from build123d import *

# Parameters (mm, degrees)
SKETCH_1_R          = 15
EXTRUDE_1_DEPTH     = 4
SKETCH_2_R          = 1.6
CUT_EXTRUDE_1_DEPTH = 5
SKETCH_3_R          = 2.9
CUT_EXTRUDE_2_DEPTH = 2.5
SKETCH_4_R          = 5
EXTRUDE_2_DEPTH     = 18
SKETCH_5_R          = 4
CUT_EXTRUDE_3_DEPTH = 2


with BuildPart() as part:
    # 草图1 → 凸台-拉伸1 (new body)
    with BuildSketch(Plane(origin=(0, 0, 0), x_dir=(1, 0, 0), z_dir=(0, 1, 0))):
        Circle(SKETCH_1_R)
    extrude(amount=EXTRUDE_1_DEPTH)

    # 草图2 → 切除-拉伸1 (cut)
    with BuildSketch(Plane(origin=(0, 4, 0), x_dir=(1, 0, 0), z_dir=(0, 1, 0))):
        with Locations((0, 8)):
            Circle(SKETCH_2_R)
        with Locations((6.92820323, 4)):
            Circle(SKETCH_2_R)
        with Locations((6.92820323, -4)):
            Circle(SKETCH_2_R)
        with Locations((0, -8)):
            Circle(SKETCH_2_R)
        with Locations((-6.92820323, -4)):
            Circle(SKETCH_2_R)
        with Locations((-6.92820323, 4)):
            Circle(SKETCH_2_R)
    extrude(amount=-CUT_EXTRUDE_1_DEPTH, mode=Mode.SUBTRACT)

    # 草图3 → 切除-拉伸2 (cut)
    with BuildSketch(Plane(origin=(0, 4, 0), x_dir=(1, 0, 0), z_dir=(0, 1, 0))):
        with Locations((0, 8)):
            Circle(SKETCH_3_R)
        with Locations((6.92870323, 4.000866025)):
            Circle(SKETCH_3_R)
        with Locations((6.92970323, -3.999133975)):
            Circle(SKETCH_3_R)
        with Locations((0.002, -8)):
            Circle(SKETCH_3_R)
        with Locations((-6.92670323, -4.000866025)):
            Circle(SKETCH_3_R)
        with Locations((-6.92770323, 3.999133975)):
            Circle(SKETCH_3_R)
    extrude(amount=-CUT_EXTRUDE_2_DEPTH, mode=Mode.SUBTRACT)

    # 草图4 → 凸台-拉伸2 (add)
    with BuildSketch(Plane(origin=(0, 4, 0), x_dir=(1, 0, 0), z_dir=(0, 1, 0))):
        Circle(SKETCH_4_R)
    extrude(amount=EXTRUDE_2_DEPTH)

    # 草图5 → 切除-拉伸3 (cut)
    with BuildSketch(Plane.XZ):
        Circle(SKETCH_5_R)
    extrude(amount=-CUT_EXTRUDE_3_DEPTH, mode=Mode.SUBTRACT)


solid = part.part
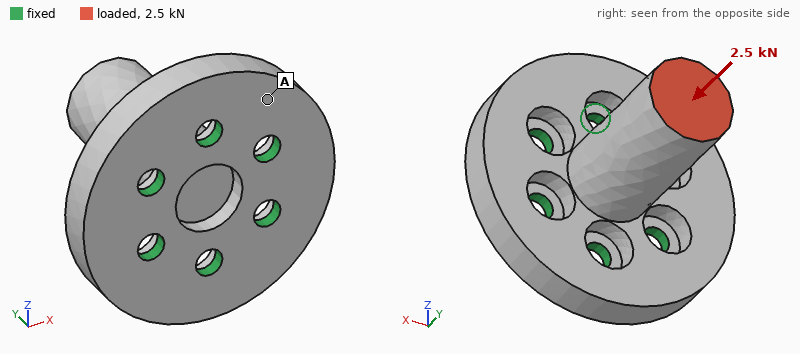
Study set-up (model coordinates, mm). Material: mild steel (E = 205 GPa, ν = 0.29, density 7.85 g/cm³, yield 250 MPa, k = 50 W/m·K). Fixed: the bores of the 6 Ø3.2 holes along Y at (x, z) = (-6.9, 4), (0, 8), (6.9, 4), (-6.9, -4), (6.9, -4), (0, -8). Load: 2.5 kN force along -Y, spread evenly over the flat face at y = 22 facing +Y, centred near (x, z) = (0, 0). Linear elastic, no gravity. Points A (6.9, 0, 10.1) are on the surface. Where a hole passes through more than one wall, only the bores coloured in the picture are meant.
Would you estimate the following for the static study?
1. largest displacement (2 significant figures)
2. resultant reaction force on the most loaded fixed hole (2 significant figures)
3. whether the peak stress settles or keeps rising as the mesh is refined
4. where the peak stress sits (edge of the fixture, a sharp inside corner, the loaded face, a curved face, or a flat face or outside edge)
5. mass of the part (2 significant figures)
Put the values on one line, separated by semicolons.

5.2 µm; 520 N; keeps rising; edge of the fixture; 29 g
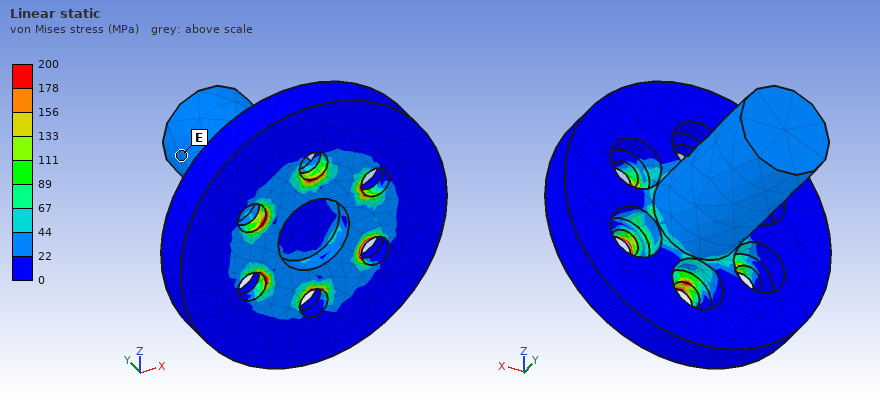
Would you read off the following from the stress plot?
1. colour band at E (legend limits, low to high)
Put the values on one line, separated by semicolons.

22 to 44 MPa
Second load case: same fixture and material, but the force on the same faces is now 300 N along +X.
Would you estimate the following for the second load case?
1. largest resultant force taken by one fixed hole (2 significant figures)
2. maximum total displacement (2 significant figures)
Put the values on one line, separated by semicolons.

280 N; 14 µm
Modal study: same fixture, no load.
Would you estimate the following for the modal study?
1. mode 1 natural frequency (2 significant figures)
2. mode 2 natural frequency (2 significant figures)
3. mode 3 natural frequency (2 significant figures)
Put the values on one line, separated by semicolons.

13 kHz; 13 kHz; 33 kHz
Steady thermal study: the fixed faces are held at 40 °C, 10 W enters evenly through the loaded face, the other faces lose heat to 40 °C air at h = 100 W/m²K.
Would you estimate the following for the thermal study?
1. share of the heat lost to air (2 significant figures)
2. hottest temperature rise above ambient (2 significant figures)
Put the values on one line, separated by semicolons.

21 %; 52 K
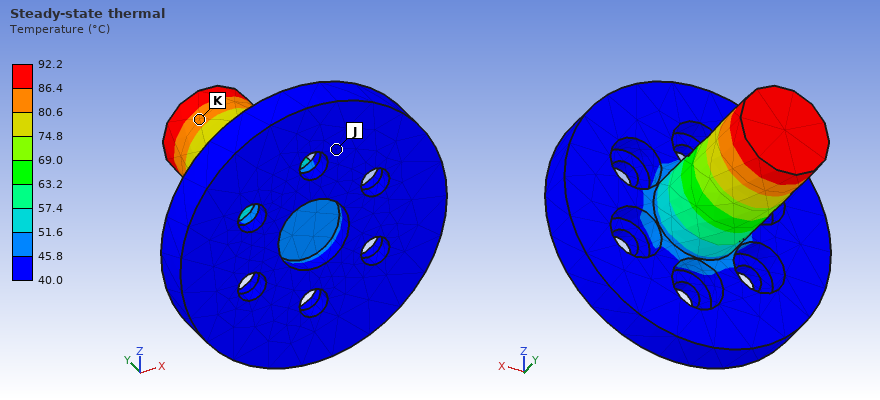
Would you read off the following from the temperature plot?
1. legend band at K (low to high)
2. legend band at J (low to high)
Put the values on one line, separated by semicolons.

80.6 to 86.4 °C; 40.0 to 45.8 °C
